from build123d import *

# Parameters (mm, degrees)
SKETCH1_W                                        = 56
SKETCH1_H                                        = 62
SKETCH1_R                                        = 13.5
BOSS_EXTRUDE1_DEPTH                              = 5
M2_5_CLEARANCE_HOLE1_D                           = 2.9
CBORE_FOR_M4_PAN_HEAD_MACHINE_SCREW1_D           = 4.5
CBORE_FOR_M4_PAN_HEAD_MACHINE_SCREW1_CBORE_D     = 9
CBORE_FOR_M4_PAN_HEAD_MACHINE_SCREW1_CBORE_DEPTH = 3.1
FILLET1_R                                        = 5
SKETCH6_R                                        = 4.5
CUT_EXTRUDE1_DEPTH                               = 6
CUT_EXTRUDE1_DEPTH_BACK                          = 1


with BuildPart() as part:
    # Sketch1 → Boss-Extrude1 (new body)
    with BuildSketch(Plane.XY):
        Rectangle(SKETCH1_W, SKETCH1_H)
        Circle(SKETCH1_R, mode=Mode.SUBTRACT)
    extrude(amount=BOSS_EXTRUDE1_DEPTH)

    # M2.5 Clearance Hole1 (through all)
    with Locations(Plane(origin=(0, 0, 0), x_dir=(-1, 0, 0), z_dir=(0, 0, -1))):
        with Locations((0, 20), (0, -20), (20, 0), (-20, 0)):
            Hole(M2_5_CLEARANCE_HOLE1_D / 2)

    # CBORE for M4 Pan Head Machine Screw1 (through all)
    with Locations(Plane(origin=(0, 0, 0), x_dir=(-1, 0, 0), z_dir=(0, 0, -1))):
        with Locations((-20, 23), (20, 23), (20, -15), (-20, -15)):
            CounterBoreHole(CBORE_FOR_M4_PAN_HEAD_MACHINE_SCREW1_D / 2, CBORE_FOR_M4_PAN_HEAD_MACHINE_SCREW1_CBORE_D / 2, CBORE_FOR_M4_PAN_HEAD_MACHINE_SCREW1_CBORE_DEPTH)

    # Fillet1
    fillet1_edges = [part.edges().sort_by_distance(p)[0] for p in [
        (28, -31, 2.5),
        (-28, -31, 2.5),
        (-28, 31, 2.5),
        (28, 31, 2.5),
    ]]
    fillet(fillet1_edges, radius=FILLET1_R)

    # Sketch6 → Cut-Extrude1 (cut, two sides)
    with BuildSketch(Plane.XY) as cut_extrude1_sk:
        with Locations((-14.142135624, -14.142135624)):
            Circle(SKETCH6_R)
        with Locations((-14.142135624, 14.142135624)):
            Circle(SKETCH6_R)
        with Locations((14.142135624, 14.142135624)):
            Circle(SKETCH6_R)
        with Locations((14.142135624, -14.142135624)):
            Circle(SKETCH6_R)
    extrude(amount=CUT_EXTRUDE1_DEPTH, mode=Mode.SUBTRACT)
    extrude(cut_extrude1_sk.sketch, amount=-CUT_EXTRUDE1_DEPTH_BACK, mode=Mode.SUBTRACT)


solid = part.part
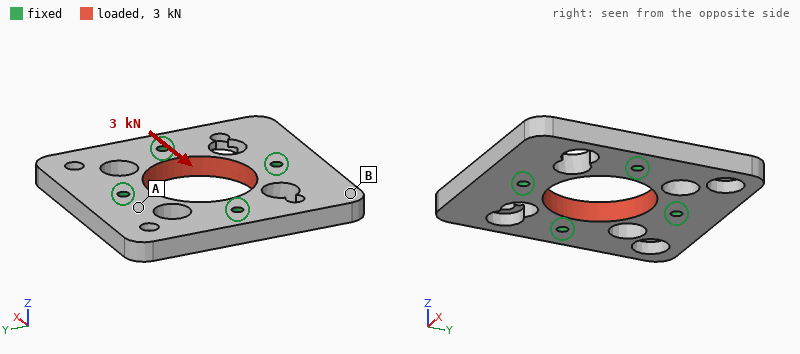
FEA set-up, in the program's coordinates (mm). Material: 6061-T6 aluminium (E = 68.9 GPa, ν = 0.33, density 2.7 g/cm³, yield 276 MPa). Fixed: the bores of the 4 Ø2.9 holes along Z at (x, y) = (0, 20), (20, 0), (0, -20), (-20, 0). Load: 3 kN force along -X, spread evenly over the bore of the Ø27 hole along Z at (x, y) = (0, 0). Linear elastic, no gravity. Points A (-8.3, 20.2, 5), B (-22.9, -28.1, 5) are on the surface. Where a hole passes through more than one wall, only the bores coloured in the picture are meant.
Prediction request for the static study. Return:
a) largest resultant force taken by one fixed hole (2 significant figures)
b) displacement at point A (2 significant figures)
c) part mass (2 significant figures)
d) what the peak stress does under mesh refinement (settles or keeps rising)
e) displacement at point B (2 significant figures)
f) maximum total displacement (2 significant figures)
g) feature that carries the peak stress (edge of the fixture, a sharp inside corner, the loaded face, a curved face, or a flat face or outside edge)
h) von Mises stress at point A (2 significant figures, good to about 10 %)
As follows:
770 N
1.4 µm
33 g
keeps rising
1.0 µm
4.6 µm
edge of the fixture
6.0 MPa
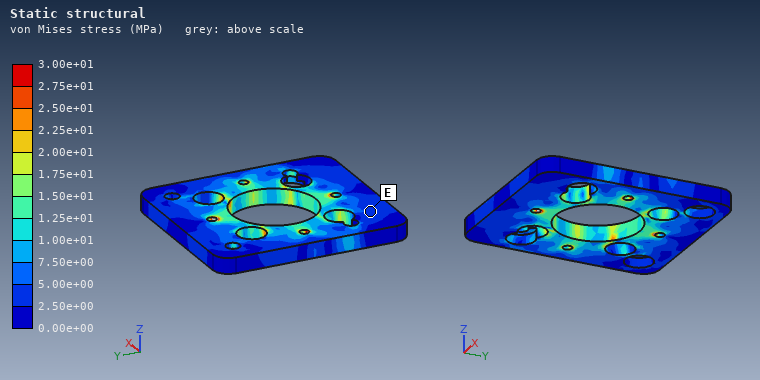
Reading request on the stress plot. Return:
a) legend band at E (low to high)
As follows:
2.50e+00 to 5.00e+00 MPa
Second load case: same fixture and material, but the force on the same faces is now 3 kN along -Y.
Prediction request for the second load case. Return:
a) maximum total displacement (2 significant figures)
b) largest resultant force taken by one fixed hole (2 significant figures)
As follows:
5.0 µm
760 N
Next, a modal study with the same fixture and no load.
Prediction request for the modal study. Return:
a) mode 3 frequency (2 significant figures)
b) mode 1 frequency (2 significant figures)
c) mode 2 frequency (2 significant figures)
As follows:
8000 Hz
7100 Hz
7800 Hz
